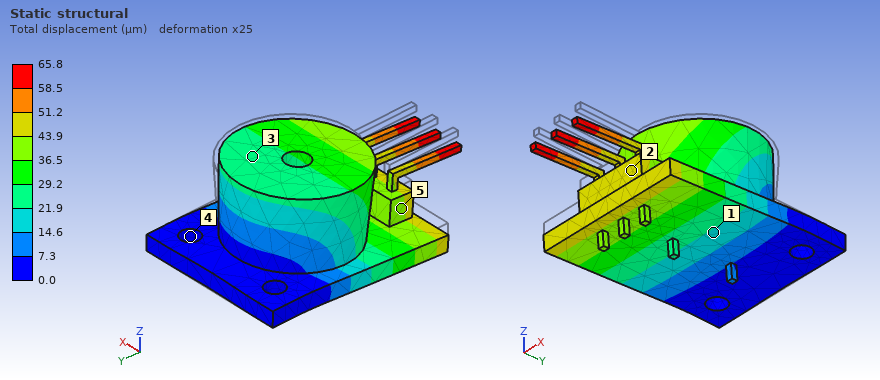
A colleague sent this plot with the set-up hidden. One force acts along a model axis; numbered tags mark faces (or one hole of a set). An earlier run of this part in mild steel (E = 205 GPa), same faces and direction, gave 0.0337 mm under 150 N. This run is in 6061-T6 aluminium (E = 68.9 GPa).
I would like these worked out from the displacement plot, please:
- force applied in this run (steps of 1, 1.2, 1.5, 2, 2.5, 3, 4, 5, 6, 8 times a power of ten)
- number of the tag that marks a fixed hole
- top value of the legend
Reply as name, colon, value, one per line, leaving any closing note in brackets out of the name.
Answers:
force applied in this run: 100 N
number of the tag that marks a fixed hole: 4
top value of the legend: 65.8 µm
